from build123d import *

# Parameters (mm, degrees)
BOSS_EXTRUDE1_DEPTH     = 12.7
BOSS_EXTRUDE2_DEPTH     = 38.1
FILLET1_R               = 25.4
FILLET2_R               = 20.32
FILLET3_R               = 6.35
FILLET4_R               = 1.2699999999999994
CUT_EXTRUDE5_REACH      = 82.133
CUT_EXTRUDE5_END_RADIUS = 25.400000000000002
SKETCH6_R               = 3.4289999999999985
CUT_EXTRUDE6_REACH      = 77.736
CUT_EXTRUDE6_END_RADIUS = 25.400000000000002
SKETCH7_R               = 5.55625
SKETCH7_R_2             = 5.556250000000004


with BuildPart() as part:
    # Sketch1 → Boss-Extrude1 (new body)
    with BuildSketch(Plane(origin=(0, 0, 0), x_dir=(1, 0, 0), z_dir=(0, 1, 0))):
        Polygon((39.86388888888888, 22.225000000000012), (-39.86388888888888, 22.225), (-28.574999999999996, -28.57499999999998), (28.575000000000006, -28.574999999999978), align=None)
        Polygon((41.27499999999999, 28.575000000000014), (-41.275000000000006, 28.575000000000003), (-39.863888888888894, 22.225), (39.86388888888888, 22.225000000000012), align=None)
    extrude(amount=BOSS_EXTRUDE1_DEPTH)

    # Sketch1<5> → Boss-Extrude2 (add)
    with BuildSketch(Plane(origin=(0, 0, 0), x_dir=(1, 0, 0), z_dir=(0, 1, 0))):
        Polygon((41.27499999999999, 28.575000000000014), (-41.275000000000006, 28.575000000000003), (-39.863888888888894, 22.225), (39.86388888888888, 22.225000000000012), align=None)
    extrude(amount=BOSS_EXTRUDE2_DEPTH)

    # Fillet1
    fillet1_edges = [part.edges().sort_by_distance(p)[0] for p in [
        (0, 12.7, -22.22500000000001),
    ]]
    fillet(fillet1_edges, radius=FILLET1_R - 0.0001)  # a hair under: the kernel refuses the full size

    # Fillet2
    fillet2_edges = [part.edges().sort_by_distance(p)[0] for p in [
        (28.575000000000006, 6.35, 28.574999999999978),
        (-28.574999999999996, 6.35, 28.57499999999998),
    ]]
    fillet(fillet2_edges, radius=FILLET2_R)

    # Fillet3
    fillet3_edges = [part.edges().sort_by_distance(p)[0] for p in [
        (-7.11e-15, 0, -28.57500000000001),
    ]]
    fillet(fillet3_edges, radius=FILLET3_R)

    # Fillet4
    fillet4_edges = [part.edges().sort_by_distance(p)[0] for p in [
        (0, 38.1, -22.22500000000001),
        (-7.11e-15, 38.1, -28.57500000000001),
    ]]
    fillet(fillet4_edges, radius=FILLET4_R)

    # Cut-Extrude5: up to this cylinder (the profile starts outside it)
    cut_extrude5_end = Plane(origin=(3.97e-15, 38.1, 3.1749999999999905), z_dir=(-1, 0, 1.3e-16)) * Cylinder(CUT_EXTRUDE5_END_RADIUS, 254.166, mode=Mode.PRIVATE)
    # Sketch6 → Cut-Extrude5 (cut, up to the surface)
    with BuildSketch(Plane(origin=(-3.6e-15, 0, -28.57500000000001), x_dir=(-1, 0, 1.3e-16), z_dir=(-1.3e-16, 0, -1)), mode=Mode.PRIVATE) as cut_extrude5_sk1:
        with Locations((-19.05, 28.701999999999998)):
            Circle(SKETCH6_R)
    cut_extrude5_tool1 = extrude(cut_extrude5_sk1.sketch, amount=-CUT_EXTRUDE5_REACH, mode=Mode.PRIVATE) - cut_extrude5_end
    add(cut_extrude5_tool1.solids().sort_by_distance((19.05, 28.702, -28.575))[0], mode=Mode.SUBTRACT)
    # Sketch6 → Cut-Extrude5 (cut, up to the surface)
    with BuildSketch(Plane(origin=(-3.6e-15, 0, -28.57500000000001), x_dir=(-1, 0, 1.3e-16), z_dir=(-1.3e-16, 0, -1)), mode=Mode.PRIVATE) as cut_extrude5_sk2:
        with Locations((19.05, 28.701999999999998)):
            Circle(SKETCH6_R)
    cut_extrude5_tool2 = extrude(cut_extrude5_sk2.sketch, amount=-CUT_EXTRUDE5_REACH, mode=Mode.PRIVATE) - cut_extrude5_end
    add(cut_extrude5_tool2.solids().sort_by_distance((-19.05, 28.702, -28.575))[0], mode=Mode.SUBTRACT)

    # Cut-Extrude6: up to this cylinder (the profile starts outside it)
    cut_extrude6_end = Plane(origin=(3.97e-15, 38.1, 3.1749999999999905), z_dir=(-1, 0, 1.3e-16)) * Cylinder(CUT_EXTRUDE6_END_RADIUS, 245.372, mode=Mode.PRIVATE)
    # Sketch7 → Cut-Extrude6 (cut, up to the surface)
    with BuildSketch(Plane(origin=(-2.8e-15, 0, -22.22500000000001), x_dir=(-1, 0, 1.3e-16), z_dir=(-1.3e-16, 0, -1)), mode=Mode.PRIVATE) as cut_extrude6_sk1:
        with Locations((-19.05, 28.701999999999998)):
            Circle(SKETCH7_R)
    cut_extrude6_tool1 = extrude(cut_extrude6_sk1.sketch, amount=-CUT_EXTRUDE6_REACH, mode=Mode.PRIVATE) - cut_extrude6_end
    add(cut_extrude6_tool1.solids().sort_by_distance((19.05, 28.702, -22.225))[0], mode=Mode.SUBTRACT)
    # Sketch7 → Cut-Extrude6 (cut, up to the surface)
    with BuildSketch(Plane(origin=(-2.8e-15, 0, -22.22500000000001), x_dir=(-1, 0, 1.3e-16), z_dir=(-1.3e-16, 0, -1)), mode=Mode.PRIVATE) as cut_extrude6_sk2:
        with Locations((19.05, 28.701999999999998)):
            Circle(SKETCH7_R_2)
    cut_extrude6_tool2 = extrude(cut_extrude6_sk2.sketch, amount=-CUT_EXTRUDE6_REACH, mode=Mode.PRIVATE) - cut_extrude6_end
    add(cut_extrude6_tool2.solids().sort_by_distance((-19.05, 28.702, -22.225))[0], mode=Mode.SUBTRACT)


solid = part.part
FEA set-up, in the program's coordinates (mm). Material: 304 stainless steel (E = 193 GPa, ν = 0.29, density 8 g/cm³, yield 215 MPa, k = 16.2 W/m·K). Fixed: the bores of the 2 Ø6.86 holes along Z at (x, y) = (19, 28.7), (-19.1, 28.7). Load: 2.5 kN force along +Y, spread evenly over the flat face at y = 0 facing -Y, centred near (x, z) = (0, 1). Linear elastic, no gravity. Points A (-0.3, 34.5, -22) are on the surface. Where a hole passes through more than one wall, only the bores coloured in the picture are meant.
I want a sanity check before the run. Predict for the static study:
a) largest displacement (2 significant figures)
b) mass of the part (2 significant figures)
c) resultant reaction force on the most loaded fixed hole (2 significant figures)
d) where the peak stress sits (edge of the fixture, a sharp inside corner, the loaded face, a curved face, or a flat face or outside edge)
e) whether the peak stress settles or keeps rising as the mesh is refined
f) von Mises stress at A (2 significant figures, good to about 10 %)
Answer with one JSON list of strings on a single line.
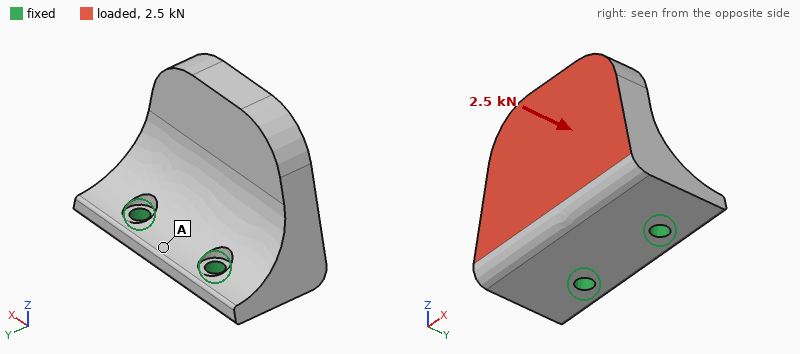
["84 µm", "570 g", "1.3 kN", "edge of the fixture", "keeps rising", "19 MPa"]
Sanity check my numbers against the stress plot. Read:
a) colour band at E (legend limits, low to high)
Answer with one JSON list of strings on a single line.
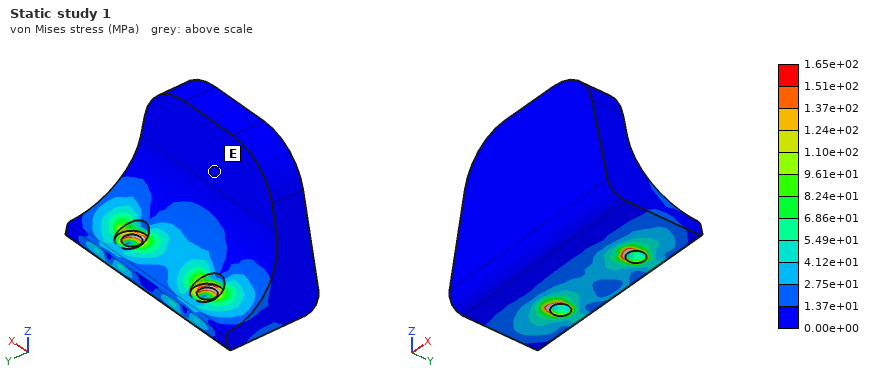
["0.00e+00 to 1.37e+01 MPa"]
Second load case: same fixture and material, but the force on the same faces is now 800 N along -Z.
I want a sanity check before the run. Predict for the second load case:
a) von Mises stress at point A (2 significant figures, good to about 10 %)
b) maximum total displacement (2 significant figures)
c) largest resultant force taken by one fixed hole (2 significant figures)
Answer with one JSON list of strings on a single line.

["5.4 MPa", "25 µm", "400 N"]
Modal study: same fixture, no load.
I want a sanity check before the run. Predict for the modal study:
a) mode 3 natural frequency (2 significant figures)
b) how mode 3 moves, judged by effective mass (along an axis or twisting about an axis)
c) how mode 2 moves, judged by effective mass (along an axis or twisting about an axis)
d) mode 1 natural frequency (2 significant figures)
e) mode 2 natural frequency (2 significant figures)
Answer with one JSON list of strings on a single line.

["7300 Hz", "along X", "along X", "1600 Hz", "4100 Hz"]
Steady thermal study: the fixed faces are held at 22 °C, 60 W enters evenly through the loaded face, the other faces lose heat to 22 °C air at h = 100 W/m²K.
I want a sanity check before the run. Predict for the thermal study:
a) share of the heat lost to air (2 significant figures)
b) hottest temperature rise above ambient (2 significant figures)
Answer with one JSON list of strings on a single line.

["68 %", "76 K"]
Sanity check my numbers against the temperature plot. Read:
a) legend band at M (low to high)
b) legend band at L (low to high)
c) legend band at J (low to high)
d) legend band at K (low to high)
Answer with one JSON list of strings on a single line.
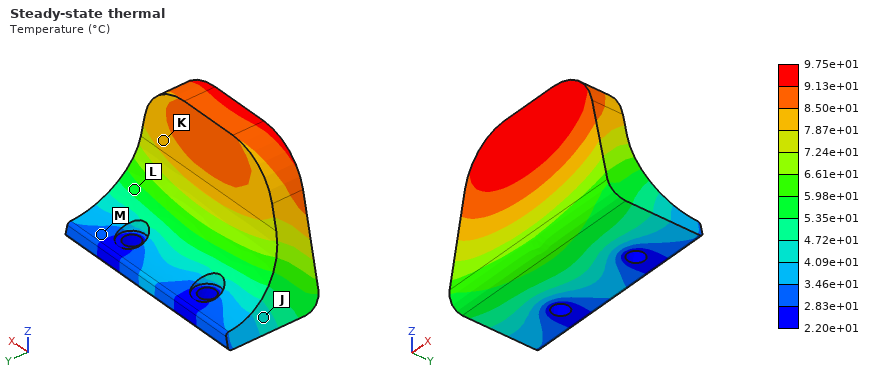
["2.83e+01 to 3.46e+01 °C", "5.35e+01 to 5.98e+01 °C", "4.09e+01 to 4.72e+01 °C", "7.87e+01 to 8.50e+01 °C"]
